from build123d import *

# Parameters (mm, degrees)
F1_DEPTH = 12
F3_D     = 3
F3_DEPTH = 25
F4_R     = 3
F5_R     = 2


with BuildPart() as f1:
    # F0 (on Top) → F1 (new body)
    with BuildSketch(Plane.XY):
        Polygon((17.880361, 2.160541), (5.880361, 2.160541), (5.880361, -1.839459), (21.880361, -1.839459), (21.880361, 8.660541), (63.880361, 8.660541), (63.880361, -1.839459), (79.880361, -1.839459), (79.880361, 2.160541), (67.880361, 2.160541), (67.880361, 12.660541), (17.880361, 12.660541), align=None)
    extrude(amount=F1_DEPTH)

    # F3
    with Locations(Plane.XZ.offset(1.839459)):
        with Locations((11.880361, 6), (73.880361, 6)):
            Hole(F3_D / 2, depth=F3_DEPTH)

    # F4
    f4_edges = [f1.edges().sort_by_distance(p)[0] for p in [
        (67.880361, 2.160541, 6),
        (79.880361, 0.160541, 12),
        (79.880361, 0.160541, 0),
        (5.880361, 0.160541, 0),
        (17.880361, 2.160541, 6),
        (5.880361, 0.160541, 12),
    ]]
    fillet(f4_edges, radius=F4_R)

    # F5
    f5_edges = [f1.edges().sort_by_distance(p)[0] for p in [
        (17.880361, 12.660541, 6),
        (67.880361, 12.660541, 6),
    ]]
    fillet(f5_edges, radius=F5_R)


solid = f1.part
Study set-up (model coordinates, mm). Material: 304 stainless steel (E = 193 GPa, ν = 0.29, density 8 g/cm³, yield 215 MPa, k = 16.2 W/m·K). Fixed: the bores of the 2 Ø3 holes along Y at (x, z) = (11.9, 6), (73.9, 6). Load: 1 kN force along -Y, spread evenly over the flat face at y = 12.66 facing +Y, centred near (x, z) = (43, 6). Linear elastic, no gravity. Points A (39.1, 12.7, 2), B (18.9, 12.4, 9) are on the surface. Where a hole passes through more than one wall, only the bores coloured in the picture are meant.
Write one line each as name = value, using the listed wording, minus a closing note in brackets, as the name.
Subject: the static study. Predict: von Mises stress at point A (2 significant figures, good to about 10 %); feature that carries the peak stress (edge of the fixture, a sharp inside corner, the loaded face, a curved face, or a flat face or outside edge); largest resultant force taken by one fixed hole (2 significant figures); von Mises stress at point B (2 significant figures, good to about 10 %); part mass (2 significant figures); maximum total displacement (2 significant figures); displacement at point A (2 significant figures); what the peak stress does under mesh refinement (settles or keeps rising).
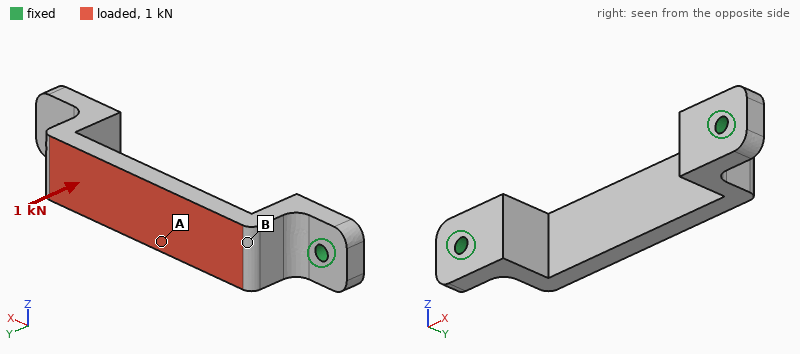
von Mises stress at point A = 74 MPa
feature that carries the peak stress = edge of the fixture
largest resultant force taken by one fixed hole = 760 N
von Mises stress at point B = 13 MPa
part mass = 36 g
maximum total displacement = 30 µm
displacement at point A = 28 µm
what the peak stress does under mesh refinement = keeps rising
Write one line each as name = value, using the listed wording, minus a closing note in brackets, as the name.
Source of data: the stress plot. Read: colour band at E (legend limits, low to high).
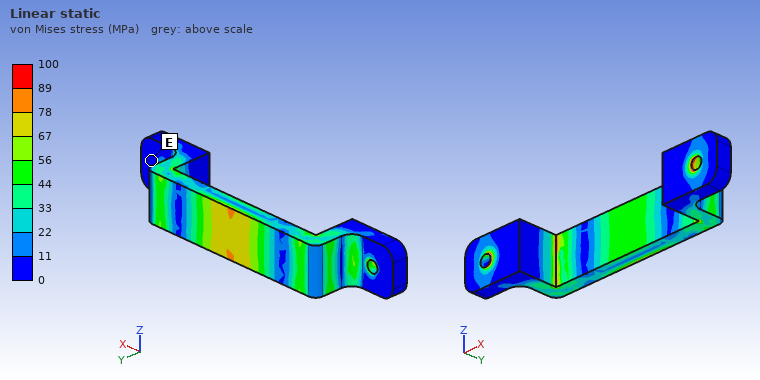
colour band at E = 0 to 11 MPa
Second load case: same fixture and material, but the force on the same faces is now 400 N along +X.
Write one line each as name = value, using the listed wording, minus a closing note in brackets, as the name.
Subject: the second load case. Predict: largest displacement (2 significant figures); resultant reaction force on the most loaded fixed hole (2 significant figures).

largest displacement = 6.8 µm
resultant reaction force on the most loaded fixed hole = 210 N
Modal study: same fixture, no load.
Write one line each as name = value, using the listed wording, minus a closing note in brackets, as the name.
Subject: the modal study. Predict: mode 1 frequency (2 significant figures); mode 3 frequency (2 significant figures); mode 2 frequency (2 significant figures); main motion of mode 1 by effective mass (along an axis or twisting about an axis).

mode 1 frequency = 6200 Hz
mode 3 frequency = 8000 Hz
mode 2 frequency = 7900 Hz
main motion of mode 1 by effective mass = along Z
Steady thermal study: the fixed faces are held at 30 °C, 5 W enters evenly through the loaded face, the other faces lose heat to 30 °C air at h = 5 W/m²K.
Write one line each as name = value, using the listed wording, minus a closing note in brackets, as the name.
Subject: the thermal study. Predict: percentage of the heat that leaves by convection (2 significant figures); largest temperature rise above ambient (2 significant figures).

percentage of the heat that leaves by convection = 8.5 %
largest temperature rise above ambient = 76 K
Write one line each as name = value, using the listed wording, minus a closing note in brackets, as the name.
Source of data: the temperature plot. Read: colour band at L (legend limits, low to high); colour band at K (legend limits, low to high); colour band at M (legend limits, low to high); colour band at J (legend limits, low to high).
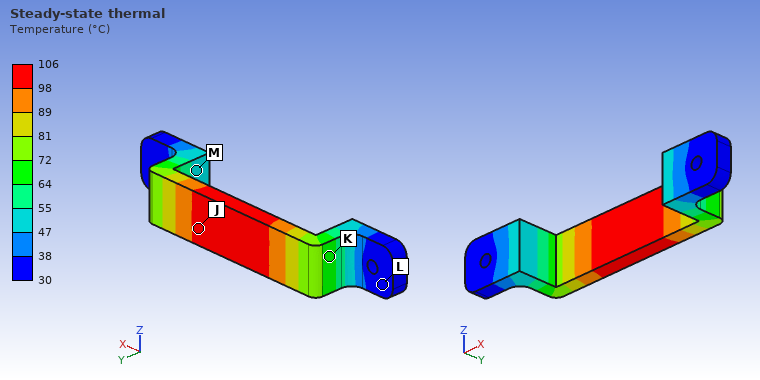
colour band at L = 30 to 38 °C
colour band at K = 64 to 72 °C
colour band at M = 47 to 55 °C
colour band at J = 98 to 106 °C
